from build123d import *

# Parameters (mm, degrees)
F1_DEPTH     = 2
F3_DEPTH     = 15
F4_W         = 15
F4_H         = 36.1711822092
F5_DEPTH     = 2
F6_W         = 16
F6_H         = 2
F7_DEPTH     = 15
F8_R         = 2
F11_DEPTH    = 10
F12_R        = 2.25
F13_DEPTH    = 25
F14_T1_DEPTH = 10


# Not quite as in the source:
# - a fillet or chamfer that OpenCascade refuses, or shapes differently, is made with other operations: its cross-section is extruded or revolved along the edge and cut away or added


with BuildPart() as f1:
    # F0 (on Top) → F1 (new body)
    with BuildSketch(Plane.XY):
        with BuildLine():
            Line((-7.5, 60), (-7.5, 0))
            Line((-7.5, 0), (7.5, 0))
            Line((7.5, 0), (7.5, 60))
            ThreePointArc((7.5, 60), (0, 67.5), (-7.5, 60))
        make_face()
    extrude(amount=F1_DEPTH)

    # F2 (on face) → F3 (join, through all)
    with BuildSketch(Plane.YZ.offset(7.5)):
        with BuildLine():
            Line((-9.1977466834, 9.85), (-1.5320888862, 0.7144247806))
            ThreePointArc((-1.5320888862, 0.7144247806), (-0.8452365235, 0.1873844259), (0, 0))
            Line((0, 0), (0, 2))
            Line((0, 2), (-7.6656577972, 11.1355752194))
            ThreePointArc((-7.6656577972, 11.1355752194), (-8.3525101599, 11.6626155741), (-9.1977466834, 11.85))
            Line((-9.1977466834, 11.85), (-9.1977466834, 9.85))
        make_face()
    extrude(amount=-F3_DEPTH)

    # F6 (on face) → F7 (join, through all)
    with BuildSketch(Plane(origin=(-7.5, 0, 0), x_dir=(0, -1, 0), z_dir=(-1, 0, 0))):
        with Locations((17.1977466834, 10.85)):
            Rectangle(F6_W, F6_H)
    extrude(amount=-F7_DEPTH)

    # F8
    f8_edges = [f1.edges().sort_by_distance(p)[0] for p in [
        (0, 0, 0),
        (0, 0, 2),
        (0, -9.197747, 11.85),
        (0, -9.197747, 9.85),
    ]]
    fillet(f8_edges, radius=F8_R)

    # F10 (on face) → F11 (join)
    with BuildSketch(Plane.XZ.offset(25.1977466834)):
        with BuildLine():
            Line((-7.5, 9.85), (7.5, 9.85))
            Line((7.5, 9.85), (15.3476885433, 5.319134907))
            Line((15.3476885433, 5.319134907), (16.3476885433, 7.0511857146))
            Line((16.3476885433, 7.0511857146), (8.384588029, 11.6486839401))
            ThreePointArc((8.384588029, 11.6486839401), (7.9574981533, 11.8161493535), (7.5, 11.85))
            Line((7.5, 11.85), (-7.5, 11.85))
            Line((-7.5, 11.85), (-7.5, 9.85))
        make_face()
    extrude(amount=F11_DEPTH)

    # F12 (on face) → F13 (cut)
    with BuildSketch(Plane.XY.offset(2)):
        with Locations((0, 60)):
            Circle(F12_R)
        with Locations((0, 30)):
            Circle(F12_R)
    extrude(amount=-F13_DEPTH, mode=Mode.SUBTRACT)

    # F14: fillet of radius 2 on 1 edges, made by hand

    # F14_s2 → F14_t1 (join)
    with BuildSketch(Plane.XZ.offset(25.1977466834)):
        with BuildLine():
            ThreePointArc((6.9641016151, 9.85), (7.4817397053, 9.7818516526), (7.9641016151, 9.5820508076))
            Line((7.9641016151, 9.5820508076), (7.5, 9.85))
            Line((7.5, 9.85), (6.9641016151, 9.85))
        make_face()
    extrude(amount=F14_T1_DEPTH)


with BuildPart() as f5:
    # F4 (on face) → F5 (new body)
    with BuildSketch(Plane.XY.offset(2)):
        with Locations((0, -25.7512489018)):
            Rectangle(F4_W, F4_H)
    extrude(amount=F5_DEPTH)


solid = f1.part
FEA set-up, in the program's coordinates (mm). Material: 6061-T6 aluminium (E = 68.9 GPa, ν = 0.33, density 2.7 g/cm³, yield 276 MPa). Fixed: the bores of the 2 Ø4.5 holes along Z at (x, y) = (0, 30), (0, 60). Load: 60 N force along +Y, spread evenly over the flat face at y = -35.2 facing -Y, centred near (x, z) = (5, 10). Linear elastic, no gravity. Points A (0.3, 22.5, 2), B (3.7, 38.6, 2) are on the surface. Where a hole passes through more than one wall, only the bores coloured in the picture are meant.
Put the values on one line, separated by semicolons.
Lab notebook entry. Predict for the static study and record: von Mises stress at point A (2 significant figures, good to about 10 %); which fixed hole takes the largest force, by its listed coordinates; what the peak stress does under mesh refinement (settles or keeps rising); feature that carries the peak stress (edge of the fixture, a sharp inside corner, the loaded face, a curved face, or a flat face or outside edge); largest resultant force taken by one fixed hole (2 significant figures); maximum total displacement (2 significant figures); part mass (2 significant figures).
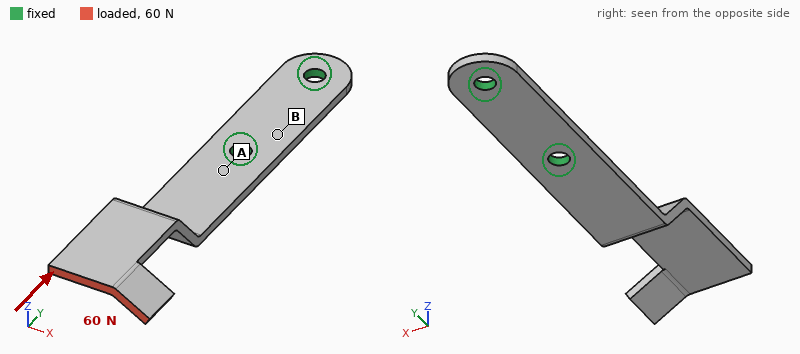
53 MPa; (0, 30); keeps rising; edge of the fixture; 56 N; 1.3 mm; 8.9 g
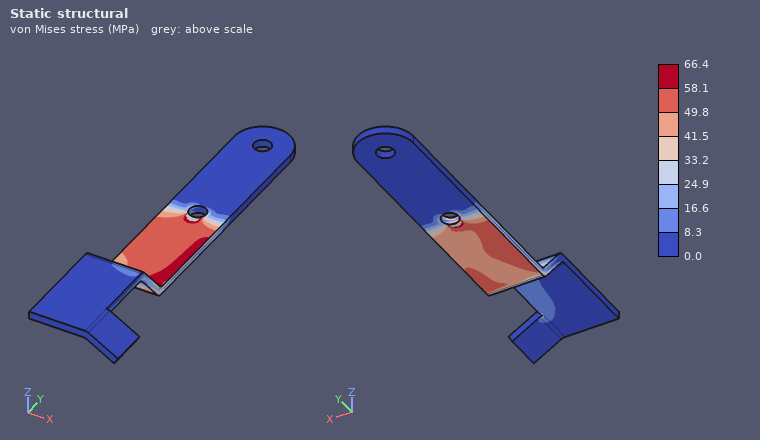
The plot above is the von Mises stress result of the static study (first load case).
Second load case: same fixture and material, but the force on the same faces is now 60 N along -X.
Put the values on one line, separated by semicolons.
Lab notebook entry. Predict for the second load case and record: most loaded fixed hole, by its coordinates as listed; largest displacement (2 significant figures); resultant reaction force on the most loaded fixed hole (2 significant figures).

(0, 30); 0.55 mm; 130 N
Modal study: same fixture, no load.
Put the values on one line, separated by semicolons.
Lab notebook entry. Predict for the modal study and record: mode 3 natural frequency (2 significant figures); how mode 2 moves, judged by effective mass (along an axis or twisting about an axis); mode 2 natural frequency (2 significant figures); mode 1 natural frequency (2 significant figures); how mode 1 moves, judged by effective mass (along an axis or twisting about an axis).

1900 Hz; along X; 1200 Hz; 330 Hz; along Z
